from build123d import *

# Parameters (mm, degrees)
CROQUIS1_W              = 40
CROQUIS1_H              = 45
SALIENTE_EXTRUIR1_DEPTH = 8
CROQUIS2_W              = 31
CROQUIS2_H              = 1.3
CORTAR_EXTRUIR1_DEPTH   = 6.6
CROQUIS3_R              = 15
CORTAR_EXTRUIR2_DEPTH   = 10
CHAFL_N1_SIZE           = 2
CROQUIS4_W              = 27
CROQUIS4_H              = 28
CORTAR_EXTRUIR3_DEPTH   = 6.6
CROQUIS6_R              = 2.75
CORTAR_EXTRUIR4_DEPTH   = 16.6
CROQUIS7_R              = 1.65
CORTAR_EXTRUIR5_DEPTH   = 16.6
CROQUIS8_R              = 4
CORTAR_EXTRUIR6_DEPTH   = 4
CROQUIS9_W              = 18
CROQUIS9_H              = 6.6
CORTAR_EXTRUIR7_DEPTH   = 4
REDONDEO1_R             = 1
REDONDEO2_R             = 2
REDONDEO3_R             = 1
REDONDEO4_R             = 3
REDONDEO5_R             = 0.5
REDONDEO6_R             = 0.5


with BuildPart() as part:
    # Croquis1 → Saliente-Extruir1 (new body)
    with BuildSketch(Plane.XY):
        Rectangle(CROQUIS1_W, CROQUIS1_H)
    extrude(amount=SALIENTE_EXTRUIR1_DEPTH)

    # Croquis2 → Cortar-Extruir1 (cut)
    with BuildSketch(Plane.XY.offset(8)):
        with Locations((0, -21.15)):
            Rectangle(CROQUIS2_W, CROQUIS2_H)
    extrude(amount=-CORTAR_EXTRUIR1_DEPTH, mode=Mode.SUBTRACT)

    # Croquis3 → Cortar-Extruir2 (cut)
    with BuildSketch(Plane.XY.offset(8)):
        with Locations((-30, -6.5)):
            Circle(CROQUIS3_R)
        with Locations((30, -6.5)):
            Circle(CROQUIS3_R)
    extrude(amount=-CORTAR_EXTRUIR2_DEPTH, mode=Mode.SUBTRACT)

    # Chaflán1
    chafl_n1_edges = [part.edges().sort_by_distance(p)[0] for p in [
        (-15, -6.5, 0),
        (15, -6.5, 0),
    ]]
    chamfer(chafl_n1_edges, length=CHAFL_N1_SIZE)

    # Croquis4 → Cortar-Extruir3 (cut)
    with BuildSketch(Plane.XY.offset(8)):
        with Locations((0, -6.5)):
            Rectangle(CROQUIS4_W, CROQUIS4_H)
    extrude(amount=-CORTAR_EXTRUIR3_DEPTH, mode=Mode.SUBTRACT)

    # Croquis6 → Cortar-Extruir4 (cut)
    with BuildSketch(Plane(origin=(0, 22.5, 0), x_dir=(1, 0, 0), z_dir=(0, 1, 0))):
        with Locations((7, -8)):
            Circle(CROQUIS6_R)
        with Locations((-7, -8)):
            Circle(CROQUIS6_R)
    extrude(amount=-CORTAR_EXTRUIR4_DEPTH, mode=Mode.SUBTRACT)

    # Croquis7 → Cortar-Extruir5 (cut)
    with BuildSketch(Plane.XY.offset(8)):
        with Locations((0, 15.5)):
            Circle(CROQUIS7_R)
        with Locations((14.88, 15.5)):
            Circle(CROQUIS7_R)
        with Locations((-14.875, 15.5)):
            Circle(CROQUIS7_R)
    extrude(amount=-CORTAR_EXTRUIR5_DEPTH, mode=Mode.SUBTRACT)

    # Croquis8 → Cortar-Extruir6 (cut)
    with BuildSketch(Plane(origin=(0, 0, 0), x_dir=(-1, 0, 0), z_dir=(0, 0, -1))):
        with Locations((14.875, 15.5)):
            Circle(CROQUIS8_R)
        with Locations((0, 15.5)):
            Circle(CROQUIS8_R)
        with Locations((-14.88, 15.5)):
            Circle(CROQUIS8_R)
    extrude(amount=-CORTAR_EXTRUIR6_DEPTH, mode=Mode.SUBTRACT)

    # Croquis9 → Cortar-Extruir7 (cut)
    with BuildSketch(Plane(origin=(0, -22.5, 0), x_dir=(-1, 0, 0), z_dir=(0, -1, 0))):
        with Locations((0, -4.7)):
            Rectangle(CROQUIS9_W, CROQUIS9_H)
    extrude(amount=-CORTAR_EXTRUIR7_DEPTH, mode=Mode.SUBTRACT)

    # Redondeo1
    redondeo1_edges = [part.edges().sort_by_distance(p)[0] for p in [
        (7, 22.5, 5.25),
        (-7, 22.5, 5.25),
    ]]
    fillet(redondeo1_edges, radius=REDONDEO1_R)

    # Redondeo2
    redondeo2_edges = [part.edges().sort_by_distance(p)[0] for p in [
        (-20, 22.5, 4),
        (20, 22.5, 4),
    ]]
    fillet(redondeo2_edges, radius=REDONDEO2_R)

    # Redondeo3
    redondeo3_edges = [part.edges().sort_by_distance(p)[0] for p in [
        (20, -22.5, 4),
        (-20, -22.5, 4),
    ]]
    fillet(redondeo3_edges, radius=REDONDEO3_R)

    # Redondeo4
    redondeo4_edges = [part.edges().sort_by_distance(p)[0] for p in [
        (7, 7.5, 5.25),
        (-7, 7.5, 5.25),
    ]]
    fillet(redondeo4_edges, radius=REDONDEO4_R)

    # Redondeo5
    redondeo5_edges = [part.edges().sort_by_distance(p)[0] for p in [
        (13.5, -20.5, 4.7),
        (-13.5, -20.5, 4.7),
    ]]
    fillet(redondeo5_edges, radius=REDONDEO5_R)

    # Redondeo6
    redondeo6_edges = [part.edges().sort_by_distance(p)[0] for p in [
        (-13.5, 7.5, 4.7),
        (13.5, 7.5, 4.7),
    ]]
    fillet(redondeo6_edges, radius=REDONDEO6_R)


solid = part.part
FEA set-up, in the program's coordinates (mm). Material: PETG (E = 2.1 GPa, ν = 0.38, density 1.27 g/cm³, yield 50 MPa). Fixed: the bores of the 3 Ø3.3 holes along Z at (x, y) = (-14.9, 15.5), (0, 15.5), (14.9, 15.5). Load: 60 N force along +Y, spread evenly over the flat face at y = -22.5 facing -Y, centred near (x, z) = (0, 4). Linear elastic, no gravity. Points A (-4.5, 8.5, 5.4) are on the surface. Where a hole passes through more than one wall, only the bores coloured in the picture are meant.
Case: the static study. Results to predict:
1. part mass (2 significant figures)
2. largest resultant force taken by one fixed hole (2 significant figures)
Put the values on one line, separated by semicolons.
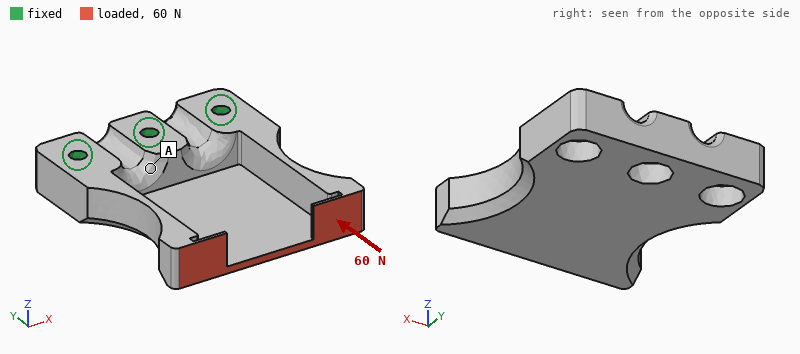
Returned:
8.4 g; 25 N
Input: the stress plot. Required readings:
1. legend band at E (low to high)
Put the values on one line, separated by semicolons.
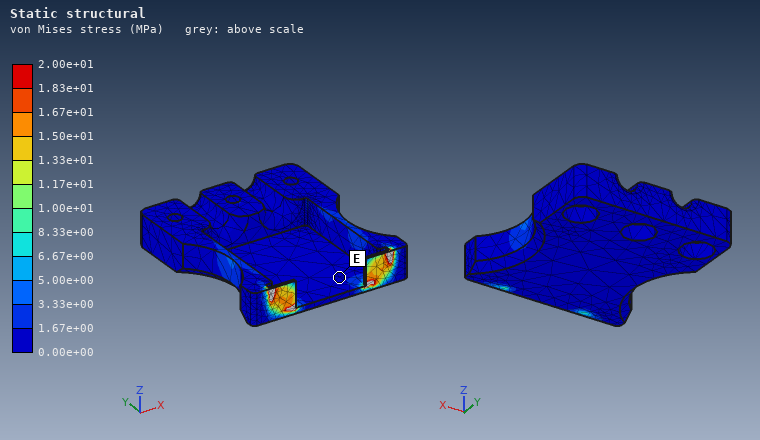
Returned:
0.00e+00 to 1.67e+00 MPa
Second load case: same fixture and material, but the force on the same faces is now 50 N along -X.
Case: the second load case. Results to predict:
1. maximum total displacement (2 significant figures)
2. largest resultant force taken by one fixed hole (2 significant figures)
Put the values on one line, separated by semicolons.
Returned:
0.67 mm; 58 N
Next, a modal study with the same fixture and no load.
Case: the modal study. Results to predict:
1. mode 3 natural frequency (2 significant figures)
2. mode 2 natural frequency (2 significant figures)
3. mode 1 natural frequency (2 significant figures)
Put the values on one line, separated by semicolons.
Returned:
1400 Hz; 930 Hz; 930 Hz
